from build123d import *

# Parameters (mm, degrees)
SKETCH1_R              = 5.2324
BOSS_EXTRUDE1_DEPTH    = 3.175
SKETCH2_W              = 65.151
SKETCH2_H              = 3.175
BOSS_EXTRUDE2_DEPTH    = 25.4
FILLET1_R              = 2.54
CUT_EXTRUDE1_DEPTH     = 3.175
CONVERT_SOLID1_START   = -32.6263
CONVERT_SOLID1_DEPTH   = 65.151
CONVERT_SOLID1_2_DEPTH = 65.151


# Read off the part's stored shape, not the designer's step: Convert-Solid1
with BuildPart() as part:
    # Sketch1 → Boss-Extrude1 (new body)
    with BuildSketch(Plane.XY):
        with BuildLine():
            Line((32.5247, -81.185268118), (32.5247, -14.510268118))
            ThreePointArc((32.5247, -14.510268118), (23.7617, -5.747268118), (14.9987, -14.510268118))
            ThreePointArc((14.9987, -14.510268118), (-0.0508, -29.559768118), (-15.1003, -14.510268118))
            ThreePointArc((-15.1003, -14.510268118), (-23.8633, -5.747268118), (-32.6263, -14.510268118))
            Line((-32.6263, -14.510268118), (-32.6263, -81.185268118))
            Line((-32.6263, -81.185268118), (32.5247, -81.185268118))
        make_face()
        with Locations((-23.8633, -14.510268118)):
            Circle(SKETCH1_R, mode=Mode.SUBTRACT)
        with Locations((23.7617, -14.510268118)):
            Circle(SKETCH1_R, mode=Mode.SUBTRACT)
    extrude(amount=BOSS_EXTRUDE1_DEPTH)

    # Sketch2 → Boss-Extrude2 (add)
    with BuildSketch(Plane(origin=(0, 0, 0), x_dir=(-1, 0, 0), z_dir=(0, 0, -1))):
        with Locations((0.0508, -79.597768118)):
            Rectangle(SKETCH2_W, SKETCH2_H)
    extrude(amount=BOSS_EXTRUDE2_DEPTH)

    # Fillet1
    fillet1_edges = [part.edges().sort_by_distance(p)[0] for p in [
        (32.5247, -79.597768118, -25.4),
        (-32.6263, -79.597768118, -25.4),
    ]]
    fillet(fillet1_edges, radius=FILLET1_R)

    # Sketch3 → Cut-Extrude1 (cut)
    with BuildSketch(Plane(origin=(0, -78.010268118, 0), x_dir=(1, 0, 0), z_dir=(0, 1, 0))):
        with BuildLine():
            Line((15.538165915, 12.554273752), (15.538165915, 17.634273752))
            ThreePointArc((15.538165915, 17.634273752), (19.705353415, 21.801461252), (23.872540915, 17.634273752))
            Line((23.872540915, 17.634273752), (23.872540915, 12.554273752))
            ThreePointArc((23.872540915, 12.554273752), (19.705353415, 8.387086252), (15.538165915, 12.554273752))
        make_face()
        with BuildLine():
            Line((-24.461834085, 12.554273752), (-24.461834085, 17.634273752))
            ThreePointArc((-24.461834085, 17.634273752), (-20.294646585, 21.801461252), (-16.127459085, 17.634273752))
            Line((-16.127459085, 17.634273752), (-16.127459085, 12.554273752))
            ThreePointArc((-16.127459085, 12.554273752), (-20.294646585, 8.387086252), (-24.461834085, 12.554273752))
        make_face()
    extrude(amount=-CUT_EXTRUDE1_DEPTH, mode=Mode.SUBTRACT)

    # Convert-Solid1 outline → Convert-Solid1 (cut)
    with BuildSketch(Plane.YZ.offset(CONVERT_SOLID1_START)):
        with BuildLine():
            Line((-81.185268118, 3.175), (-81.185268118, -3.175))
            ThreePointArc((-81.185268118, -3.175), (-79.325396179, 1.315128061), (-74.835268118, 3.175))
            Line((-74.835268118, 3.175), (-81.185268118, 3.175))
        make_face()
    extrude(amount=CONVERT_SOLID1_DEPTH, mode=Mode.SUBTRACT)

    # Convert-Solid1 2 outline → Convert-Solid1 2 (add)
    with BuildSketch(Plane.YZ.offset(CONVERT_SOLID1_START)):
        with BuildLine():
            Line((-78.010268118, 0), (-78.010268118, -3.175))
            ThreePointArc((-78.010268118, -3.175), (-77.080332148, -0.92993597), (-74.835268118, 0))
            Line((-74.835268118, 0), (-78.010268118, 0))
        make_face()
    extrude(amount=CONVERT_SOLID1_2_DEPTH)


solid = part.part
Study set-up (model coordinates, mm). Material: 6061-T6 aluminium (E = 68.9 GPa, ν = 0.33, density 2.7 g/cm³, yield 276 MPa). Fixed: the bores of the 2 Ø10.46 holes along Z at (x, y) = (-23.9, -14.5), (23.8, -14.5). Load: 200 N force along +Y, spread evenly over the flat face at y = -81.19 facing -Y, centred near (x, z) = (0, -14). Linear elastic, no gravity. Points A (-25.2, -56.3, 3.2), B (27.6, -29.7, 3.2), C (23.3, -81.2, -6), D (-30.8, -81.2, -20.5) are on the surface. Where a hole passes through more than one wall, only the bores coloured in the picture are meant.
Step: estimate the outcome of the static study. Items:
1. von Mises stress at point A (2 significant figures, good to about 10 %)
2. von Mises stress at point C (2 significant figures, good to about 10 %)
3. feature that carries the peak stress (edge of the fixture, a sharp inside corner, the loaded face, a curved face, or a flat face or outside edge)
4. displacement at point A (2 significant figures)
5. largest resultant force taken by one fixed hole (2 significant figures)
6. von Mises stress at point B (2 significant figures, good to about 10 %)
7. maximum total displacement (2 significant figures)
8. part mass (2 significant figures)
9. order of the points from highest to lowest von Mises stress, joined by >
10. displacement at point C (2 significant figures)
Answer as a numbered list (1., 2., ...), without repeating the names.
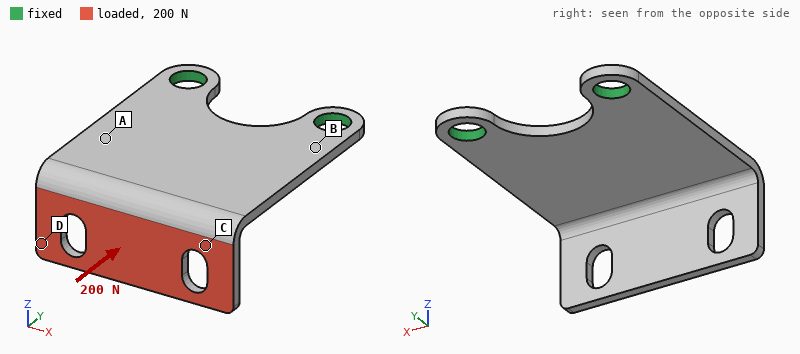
1. 28 MPa
2. 12 MPa
3. a flat face or outside edge
4. 0.24 mm
5. 100 N
6. 37 MPa
7. 0.80 mm
8. 46 g
9. B > A > C > D
10. 0.63 mm
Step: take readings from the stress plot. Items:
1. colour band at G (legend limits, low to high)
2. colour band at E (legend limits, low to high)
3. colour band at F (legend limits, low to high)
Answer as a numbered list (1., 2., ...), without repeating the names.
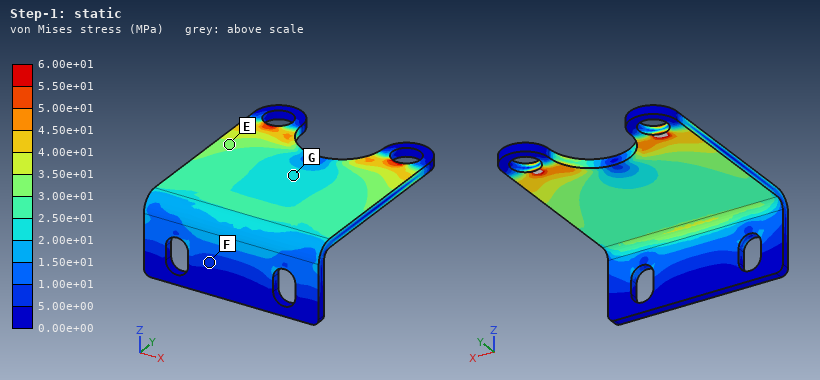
1. 2.00e+01 to 2.50e+01 MPa
2. 3.00e+01 to 3.50e+01 MPa
3. 5.00e+00 to 1.00e+01 MPa
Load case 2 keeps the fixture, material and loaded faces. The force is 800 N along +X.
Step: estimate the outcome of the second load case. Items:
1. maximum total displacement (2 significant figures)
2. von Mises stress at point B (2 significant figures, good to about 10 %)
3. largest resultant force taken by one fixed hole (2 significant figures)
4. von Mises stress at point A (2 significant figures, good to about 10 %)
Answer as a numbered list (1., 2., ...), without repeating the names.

1. 1.2 mm
2. 88 MPa
3. 1.1 kN
4. 78 MPa
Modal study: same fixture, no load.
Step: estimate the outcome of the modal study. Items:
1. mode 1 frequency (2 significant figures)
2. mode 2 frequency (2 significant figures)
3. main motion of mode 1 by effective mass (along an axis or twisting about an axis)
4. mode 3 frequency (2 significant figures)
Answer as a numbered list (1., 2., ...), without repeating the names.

1. 370 Hz
2. 990 Hz
3. along Z
4. 1900 Hz
